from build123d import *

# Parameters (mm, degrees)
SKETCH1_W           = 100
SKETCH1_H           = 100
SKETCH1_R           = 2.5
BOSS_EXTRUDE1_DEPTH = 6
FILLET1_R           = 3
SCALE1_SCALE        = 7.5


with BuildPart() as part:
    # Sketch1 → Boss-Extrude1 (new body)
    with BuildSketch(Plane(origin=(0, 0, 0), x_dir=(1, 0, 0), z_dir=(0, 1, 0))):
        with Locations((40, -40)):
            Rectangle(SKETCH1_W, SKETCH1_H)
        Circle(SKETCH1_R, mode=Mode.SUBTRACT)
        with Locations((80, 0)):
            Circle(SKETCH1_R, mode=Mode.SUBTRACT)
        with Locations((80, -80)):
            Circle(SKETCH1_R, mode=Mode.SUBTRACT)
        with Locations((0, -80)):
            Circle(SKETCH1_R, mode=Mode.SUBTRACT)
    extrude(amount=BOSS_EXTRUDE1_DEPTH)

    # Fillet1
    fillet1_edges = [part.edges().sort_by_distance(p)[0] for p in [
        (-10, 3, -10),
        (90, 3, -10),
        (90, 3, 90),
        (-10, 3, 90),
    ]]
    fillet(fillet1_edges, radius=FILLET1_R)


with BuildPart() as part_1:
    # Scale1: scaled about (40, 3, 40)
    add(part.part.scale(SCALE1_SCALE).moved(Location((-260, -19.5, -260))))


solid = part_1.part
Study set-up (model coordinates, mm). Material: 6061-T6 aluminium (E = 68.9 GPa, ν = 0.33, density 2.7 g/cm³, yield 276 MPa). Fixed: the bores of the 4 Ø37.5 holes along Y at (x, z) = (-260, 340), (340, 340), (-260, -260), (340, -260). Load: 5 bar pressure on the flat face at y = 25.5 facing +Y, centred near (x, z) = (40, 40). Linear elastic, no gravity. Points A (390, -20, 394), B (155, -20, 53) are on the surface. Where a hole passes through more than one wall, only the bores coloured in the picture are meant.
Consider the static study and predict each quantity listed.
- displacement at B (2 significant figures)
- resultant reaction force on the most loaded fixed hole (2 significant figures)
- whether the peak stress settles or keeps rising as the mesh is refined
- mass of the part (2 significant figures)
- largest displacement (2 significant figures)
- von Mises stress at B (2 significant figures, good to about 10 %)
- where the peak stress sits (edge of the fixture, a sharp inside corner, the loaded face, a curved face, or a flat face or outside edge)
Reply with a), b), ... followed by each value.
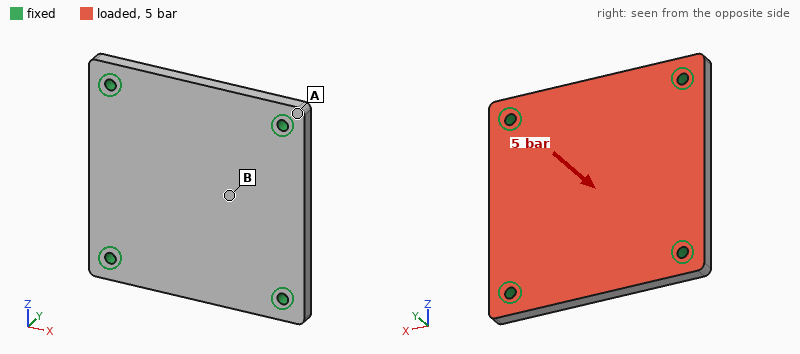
a) 0.79 mm
b) 70 kN
c) keeps rising
d) 68 kg
e) 0.87 mm
f) 27 MPa
g) edge of the fixture
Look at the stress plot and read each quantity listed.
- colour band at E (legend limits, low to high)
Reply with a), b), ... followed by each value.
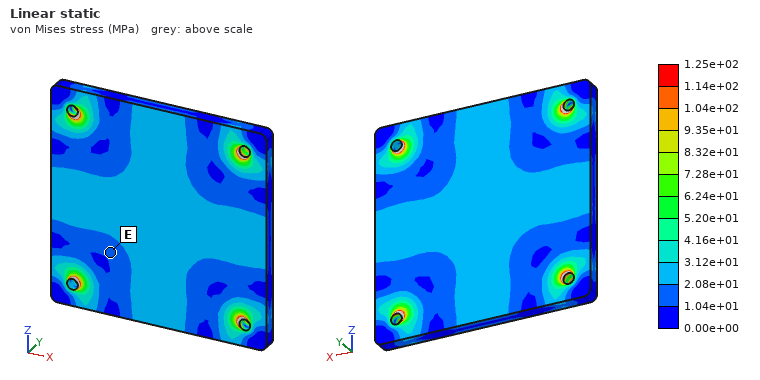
a) 1.04e+01 to 2.08e+01 MPa
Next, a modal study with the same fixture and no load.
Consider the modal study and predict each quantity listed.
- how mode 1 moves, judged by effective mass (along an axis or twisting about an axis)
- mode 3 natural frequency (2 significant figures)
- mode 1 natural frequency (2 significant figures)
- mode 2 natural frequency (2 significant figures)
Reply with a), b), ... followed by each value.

a) along Y
b) 680 Hz
c) 420 Hz
d) 680 Hz
